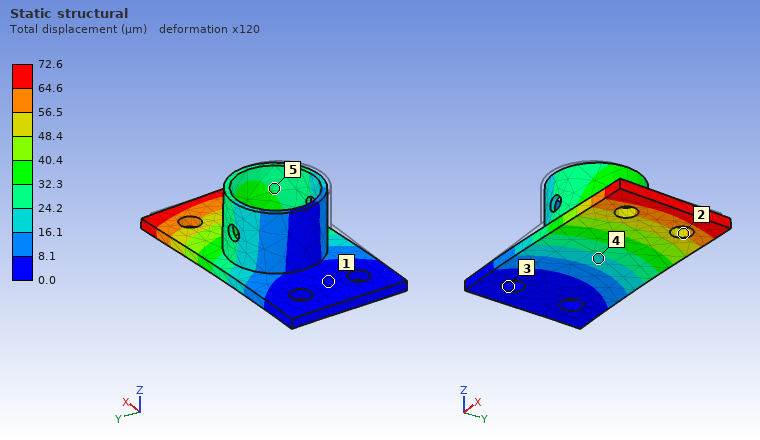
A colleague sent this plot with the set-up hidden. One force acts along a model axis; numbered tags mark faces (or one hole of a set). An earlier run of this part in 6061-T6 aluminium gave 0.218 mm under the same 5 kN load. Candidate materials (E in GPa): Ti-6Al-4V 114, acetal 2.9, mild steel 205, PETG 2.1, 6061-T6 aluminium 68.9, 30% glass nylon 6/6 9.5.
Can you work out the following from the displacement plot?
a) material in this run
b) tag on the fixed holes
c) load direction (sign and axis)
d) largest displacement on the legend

mild steel
3
+Y
72.6 µm
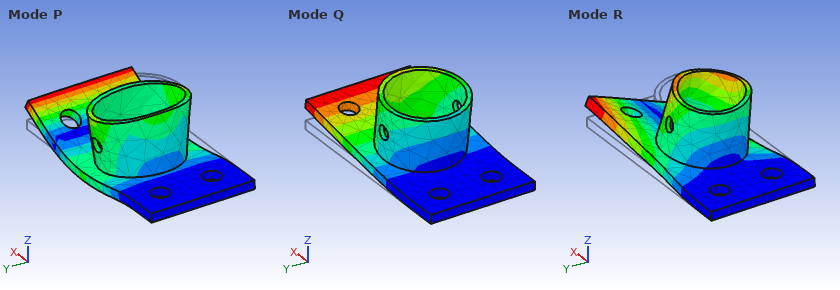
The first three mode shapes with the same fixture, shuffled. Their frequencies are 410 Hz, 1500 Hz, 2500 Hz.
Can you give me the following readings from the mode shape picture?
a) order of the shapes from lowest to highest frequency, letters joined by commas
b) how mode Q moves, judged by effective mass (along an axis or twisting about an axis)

Q, R, P
along Z
